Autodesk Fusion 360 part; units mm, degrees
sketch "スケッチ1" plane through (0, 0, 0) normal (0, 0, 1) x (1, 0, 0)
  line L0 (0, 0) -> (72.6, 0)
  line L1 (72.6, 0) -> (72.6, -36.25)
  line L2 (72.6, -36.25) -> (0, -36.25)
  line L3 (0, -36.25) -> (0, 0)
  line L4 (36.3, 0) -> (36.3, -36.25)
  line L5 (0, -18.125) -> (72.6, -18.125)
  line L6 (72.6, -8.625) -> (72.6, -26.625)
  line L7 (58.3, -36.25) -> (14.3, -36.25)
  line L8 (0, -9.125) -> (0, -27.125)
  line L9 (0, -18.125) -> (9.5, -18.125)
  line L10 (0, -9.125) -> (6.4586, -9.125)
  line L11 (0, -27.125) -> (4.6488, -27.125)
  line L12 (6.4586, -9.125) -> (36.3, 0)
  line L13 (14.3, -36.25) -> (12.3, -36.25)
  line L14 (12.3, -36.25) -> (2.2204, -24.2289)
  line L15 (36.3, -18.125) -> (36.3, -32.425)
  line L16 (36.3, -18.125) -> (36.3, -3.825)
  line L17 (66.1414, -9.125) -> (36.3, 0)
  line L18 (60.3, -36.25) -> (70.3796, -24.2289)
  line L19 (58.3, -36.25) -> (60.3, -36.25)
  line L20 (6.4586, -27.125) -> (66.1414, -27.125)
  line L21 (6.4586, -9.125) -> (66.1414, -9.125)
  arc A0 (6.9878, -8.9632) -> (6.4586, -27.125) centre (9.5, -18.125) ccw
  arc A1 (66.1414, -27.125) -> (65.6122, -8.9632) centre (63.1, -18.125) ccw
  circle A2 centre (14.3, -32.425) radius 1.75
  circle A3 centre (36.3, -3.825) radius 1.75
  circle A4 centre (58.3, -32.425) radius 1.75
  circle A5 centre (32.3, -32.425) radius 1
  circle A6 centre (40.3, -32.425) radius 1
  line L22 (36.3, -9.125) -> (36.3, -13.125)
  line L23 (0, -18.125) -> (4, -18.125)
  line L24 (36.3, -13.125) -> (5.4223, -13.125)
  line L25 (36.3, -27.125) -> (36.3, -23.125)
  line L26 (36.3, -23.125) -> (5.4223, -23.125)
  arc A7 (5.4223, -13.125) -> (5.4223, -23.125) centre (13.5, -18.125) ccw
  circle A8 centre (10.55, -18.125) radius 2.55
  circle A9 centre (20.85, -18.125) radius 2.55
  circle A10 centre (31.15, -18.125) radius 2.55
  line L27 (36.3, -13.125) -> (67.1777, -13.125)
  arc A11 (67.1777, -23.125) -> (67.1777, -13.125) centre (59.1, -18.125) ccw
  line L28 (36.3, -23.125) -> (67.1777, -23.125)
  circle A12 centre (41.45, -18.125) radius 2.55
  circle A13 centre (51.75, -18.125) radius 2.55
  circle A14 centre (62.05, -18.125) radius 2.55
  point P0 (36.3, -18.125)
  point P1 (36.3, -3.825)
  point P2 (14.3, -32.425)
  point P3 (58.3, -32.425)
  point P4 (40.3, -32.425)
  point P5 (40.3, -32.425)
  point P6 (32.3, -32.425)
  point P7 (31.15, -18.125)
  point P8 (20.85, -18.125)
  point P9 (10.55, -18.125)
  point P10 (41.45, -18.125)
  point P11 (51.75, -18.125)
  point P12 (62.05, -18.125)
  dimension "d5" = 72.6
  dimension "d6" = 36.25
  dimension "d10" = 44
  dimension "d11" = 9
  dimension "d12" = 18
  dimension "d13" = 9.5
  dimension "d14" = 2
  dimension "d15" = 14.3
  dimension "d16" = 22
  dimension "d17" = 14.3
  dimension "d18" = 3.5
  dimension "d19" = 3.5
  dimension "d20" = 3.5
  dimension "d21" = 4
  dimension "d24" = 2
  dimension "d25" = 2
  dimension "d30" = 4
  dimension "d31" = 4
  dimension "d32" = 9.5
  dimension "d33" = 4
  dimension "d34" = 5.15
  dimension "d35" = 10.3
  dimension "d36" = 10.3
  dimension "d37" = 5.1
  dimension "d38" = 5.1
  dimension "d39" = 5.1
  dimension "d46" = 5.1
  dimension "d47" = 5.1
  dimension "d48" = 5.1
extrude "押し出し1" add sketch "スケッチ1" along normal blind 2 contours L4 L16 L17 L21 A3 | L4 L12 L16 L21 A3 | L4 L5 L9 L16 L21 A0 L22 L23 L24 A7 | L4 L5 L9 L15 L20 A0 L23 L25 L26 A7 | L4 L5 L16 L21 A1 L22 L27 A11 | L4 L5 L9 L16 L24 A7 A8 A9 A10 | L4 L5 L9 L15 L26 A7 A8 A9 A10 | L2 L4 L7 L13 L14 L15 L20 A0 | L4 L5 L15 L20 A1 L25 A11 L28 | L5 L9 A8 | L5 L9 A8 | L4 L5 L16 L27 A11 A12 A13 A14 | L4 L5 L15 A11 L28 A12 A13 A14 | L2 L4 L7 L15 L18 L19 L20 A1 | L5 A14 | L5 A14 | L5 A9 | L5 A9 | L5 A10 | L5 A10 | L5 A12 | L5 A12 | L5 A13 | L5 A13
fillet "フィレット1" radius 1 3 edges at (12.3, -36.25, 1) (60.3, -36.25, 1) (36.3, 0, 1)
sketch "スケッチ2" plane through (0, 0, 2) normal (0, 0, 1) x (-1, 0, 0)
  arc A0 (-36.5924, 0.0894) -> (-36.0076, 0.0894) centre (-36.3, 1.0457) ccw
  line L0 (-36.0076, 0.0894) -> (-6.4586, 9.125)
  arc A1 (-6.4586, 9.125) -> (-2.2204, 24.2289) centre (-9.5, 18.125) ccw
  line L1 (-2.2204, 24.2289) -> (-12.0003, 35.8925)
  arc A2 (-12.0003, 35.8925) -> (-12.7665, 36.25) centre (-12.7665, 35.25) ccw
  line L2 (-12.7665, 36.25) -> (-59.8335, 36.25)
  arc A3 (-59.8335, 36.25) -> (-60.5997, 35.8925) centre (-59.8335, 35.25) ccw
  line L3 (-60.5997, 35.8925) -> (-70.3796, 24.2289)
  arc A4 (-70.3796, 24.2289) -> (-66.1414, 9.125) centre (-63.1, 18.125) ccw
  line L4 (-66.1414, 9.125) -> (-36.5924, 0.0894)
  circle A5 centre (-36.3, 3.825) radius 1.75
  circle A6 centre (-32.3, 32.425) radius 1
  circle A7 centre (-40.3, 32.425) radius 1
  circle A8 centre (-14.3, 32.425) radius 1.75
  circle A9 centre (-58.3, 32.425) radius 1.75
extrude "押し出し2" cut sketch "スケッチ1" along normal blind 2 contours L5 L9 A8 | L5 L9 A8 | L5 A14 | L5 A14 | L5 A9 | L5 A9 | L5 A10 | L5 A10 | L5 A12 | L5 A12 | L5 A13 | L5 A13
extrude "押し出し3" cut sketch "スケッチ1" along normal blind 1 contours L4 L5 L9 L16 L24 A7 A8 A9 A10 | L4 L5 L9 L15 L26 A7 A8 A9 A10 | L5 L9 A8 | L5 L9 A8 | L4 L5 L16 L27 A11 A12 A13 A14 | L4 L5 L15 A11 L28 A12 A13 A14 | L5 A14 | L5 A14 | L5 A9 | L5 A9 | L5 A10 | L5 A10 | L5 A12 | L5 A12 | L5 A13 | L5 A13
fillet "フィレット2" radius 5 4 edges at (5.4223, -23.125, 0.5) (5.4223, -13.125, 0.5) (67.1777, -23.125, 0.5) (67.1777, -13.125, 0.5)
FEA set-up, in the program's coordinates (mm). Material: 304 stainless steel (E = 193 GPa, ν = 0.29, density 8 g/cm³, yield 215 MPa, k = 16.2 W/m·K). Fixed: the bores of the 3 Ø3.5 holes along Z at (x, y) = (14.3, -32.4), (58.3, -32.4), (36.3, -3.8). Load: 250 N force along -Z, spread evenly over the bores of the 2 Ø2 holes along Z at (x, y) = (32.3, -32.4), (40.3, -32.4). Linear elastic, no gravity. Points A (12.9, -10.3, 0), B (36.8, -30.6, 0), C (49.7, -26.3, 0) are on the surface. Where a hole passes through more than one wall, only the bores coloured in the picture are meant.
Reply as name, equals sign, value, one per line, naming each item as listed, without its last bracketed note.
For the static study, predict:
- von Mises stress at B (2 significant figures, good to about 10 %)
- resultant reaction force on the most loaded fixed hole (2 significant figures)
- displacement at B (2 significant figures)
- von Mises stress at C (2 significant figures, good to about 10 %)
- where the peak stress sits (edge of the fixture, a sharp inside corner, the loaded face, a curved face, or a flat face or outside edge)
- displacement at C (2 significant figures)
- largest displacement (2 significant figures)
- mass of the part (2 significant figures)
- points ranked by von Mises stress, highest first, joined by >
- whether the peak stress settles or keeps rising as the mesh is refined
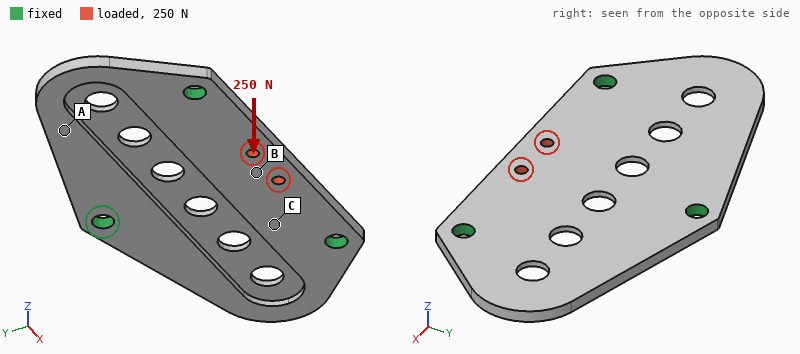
von Mises stress at B = 74 MPa
resultant reaction force on the most loaded fixed hole = 120 N
displacement at B = 50 µm
von Mises stress at C = 49 MPa
where the peak stress sits = edge of the fixture
displacement at C = 13 µm
largest displacement = 65 µm
mass of the part = 26 g
points ranked by von Mises stress, highest first, joined by > = B > C > A
whether the peak stress settles or keeps rising as the mesh is refined = keeps rising
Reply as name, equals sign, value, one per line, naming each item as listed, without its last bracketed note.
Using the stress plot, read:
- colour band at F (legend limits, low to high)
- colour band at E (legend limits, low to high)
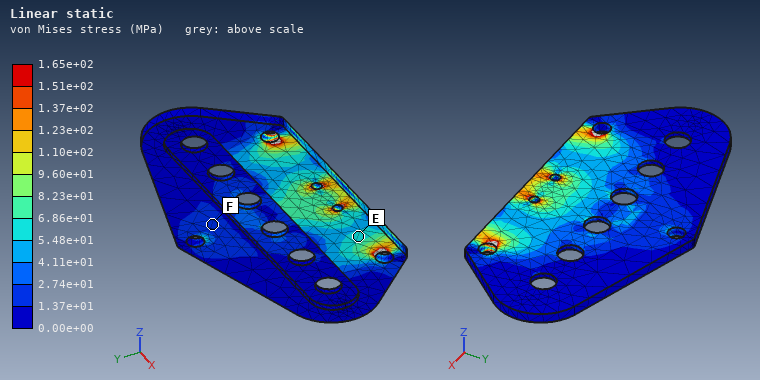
colour band at F = 1.37e+01 to 2.74e+01 MPa
colour band at E = 5.48e+01 to 6.86e+01 MPa
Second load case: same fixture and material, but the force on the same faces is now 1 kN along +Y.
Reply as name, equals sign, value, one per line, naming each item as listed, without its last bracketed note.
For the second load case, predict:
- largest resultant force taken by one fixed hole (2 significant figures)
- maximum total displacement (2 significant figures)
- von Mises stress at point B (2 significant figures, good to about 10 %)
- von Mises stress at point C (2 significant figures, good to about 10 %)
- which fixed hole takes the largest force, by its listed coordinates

largest resultant force taken by one fixed hole = 400 N
maximum total displacement = 7.4 µm
von Mises stress at point B = 11 MPa
von Mises stress at point C = 28 MPa
which fixed hole takes the largest force, by its listed coordinates = (36.3, -3.8)
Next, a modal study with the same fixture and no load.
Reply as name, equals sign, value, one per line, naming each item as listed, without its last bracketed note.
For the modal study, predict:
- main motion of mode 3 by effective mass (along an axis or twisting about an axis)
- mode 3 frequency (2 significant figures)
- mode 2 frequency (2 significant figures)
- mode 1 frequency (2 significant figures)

main motion of mode 3 by effective mass = along Z
mode 3 frequency = 5800 Hz
mode 2 frequency = 3600 Hz
mode 1 frequency = 3600 Hz
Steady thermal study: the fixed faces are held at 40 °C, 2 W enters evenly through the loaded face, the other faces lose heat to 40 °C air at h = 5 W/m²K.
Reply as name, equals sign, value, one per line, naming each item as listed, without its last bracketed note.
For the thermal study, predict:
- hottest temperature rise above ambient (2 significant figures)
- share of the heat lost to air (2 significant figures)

hottest temperature rise above ambient = 41 K
share of the heat lost to air = 10 %
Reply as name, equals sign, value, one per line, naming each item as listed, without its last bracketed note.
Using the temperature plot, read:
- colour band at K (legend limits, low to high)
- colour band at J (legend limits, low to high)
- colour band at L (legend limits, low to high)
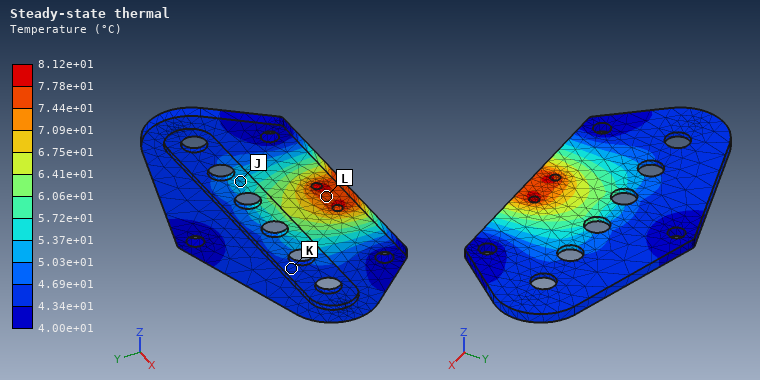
colour band at K = 4.34e+01 to 4.69e+01 °C
colour band at J = 5.03e+01 to 5.37e+01 °C
colour band at L = 7.44e+01 to 7.78e+01 °C
